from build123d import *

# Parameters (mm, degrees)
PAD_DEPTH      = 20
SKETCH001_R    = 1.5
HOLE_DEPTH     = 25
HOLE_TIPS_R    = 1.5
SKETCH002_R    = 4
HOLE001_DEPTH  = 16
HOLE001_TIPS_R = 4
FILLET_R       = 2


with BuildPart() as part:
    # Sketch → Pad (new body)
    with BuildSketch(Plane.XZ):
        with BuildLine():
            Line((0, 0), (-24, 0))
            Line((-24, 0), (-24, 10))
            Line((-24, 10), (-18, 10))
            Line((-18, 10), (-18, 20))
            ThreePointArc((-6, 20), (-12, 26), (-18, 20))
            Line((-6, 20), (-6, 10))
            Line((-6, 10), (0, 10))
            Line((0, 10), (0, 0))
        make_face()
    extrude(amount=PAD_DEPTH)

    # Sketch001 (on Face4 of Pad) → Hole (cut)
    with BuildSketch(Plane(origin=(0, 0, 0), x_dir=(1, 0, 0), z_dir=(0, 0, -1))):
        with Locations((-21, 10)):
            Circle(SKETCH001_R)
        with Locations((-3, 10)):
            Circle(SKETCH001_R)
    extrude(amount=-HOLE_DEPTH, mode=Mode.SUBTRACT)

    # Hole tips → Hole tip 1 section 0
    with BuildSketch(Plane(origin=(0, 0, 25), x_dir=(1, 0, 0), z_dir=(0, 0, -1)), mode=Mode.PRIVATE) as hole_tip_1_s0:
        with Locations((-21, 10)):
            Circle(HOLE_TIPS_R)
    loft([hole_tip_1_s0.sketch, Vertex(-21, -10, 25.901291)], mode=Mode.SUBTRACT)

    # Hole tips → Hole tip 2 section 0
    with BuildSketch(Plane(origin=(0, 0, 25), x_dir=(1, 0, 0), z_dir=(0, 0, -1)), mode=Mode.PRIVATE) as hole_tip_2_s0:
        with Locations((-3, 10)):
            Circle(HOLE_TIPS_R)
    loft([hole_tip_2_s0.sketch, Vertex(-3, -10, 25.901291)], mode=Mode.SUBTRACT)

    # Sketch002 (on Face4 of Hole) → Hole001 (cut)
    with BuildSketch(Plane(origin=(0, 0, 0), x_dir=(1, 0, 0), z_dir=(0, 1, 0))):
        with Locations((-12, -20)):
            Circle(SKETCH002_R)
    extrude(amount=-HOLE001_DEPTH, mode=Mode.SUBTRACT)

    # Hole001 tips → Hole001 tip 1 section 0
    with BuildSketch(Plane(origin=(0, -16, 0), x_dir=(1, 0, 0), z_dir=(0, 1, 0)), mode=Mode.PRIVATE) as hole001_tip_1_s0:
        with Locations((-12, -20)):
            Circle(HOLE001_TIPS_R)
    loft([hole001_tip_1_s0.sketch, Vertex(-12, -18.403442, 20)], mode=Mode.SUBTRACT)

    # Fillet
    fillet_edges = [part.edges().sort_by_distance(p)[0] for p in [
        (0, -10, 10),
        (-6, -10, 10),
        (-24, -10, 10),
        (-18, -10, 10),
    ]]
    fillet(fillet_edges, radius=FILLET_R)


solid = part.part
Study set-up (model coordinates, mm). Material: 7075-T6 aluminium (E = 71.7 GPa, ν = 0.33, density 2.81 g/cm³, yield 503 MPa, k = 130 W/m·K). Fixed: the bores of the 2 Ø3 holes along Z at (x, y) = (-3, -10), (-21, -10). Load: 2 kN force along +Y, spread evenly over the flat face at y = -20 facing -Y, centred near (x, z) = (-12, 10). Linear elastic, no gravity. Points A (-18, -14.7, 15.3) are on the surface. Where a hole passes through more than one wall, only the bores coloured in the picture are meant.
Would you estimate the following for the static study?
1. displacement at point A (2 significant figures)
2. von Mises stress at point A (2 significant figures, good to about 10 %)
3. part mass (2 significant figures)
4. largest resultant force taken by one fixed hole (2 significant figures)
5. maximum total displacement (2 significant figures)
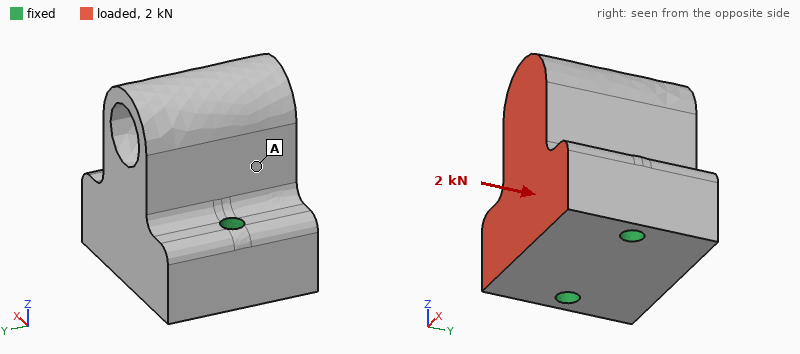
6.0 µm
8.6 MPa
21 g
1.0 kN
13 µm
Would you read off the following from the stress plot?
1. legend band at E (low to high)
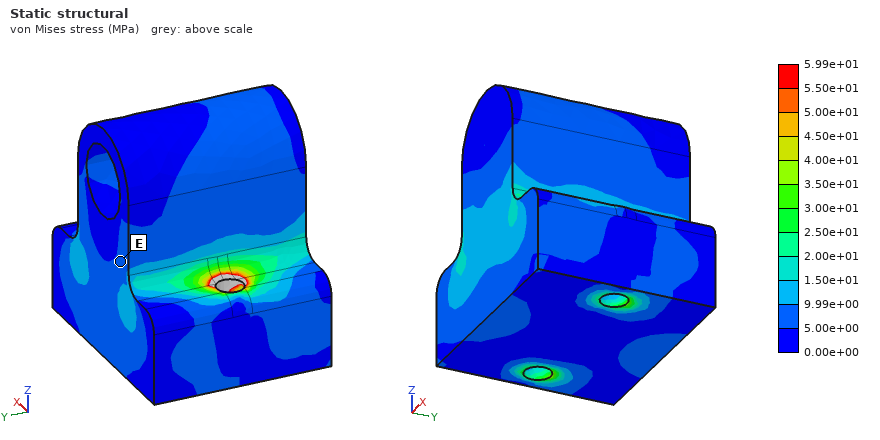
5.00e+00 to 9.99e+00 MPa
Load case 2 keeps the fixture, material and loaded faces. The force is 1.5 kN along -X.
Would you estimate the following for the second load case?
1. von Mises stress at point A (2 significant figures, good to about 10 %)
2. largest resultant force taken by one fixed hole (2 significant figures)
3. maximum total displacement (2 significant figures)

13 MPa
1.1 kN
9.2 µm
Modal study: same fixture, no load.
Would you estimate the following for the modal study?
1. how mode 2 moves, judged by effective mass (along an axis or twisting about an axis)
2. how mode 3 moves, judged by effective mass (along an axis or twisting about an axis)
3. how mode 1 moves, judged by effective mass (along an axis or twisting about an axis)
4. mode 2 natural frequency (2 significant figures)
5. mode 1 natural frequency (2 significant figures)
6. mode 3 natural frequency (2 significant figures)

along X
along Z
along Y
24 kHz
18 kHz
38 kHz
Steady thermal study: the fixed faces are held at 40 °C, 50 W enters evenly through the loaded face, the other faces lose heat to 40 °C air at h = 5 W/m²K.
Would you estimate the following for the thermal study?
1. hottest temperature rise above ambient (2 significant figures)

23 K
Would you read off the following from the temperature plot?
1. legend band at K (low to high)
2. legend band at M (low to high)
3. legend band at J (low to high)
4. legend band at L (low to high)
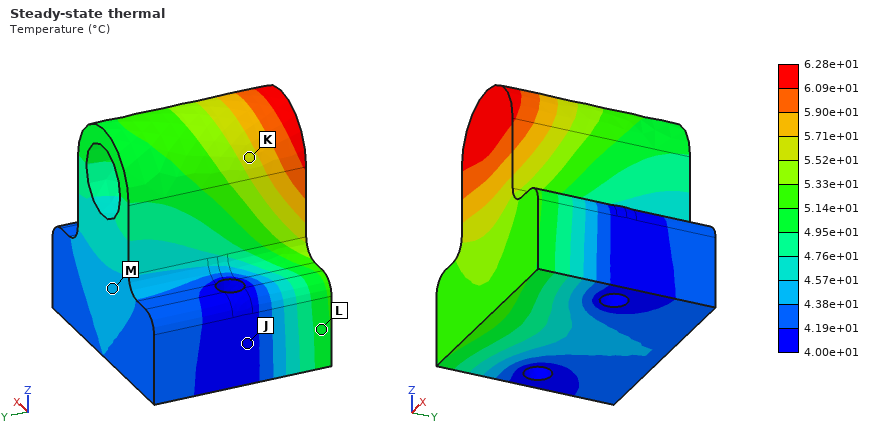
5.52e+01 to 5.71e+01 °C
4.38e+01 to 4.57e+01 °C
4.00e+01 to 4.19e+01 °C
4.95e+01 to 5.14e+01 °C
